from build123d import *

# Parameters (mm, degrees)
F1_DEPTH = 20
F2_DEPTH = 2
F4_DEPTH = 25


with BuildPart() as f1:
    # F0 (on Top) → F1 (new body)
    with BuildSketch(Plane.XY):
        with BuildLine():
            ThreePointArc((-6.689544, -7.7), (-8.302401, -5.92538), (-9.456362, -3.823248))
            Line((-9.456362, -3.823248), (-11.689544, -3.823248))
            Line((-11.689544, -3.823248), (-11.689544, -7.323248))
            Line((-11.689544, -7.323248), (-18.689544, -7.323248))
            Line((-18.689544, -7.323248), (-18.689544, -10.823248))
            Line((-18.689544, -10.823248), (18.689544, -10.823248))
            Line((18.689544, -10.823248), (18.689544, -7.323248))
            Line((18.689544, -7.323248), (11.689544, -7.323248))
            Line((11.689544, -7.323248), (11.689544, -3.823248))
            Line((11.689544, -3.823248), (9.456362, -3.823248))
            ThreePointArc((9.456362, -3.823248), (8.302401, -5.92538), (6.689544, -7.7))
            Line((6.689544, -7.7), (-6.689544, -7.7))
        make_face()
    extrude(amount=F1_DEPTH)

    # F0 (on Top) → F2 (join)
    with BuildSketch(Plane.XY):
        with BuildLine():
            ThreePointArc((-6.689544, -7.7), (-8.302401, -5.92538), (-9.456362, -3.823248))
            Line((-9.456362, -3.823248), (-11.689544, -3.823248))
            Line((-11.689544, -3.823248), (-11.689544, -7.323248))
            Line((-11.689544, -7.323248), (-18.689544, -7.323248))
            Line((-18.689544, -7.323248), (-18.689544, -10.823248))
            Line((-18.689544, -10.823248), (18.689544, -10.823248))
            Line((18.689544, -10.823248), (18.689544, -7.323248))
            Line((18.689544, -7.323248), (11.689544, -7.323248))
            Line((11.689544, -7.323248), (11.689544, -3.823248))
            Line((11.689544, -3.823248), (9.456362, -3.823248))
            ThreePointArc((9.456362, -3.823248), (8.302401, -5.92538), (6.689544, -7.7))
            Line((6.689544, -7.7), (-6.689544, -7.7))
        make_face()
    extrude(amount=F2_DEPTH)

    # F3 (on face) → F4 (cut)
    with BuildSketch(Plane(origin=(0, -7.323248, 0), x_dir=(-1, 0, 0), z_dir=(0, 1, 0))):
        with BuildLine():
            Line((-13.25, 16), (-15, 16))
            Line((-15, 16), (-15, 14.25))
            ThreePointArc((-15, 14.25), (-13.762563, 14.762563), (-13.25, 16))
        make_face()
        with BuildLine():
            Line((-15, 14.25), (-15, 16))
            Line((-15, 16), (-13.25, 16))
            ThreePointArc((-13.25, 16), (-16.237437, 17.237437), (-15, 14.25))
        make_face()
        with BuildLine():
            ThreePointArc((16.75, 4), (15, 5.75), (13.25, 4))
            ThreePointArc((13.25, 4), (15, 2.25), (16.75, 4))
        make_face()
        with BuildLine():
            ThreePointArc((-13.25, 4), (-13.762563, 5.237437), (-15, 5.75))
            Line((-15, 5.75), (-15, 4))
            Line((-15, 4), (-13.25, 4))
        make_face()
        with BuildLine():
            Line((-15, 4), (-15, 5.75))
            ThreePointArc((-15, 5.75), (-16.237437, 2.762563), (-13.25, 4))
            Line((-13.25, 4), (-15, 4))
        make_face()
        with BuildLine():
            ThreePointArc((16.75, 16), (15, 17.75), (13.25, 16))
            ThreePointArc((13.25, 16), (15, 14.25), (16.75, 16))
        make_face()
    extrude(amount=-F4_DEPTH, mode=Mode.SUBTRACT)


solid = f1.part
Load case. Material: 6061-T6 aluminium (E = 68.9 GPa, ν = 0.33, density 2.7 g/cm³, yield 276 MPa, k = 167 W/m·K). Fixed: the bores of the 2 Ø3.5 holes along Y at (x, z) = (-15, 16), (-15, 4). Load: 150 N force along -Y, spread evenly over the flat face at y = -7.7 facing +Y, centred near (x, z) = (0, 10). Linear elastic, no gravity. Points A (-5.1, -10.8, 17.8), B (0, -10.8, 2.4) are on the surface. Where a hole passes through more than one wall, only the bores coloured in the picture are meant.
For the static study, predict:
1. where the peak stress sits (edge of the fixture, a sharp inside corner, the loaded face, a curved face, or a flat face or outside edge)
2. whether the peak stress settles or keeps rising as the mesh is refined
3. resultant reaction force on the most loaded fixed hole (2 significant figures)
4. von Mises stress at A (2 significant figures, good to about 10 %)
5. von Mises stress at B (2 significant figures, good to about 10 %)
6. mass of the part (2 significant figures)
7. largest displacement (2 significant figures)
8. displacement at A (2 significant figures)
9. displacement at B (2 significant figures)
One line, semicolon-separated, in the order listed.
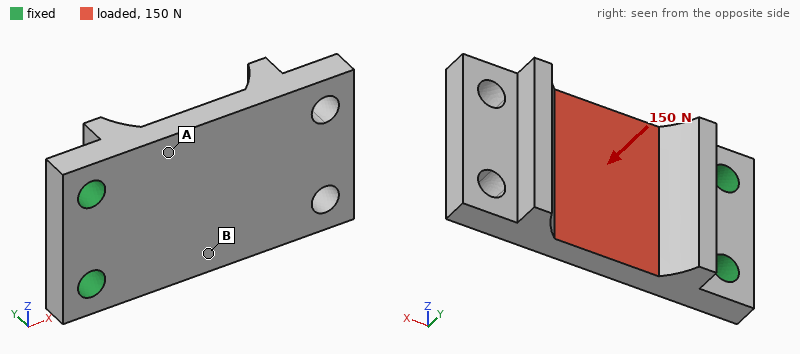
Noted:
edge of the fixture; keeps rising; 76 N; 23 MPa; 8.2 MPa; 7.6 g; 88 µm; 14 µm; 28 µm
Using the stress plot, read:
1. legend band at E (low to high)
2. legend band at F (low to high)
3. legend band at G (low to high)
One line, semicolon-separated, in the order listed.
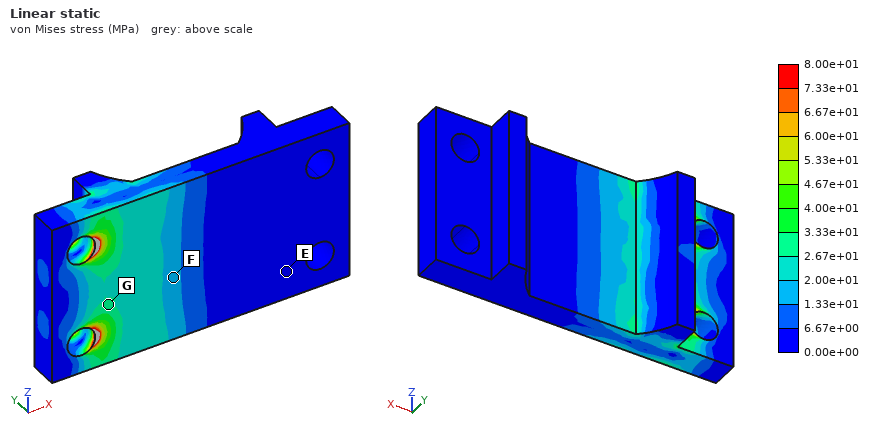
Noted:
0.00e+00 to 6.67e+00 MPa; 1.33e+01 to 2.00e+01 MPa; 2.67e+01 to 3.33e+01 MPa
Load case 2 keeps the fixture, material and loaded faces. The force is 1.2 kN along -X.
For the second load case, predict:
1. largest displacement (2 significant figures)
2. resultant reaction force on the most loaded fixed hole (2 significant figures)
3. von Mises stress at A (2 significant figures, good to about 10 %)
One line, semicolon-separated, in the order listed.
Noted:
0.13 mm; 600 N; 30 MPa
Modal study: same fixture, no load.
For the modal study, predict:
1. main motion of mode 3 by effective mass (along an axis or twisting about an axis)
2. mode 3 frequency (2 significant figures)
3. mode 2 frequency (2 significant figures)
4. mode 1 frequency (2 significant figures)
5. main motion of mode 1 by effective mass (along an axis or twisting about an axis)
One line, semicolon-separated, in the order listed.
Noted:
along Z; 11 kHz; 8400 Hz; 2500 Hz; along Y
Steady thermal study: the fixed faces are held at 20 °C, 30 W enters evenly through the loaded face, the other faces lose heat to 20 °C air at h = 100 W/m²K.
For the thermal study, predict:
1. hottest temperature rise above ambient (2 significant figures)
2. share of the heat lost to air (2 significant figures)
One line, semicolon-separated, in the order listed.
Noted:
32 K; 13 %
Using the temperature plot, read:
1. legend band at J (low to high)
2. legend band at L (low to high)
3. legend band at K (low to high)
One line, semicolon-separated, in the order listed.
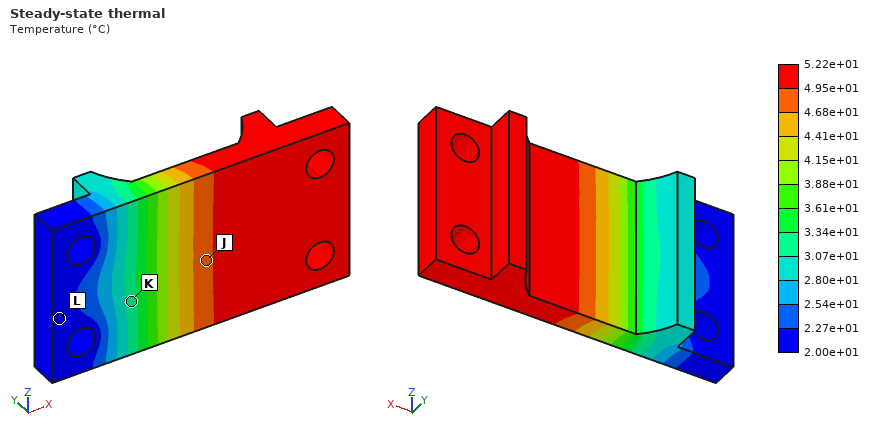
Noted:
4.68e+01 to 4.95e+01 °C; 2.00e+01 to 2.27e+01 °C; 3.07e+01 to 3.34e+01 °C
